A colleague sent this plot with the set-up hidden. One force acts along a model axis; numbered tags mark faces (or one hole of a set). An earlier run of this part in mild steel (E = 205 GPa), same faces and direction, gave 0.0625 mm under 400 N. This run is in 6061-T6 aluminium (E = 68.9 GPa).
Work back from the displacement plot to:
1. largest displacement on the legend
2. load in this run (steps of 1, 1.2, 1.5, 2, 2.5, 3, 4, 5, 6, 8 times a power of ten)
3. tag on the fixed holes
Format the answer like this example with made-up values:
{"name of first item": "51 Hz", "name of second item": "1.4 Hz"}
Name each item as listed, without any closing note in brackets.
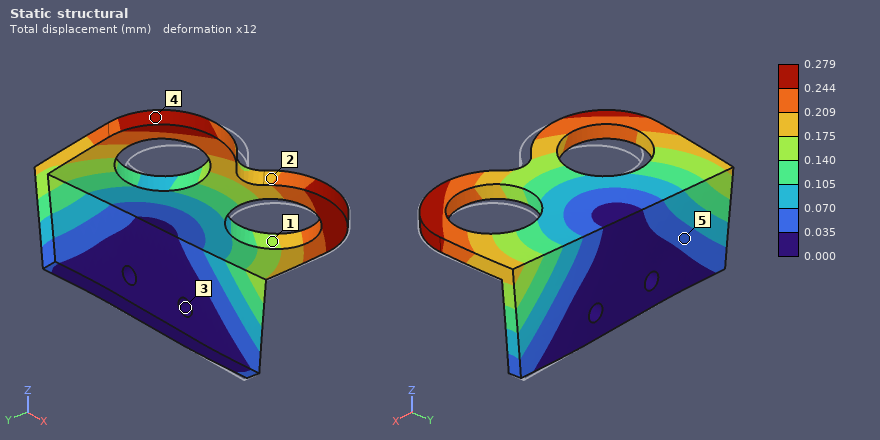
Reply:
{"largest displacement on the legend": "0.279 mm", "load in this run": "600 N", "tag on the fixed holes": "3"}
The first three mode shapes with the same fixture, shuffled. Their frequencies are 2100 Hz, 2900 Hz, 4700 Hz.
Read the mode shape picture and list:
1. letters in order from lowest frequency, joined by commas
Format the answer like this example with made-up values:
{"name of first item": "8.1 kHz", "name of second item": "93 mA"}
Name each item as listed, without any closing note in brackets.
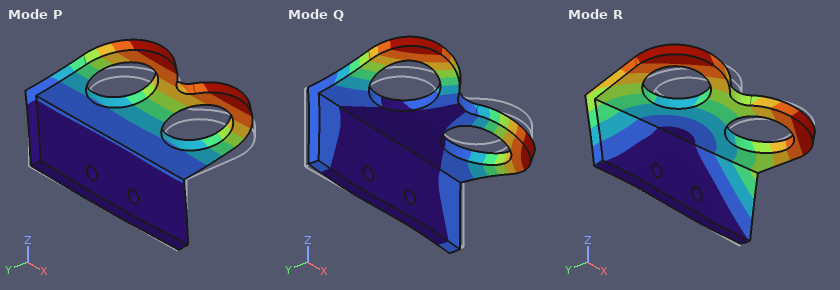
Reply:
{"letters in order from lowest frequency, joined by commas": "P, R, Q"}
